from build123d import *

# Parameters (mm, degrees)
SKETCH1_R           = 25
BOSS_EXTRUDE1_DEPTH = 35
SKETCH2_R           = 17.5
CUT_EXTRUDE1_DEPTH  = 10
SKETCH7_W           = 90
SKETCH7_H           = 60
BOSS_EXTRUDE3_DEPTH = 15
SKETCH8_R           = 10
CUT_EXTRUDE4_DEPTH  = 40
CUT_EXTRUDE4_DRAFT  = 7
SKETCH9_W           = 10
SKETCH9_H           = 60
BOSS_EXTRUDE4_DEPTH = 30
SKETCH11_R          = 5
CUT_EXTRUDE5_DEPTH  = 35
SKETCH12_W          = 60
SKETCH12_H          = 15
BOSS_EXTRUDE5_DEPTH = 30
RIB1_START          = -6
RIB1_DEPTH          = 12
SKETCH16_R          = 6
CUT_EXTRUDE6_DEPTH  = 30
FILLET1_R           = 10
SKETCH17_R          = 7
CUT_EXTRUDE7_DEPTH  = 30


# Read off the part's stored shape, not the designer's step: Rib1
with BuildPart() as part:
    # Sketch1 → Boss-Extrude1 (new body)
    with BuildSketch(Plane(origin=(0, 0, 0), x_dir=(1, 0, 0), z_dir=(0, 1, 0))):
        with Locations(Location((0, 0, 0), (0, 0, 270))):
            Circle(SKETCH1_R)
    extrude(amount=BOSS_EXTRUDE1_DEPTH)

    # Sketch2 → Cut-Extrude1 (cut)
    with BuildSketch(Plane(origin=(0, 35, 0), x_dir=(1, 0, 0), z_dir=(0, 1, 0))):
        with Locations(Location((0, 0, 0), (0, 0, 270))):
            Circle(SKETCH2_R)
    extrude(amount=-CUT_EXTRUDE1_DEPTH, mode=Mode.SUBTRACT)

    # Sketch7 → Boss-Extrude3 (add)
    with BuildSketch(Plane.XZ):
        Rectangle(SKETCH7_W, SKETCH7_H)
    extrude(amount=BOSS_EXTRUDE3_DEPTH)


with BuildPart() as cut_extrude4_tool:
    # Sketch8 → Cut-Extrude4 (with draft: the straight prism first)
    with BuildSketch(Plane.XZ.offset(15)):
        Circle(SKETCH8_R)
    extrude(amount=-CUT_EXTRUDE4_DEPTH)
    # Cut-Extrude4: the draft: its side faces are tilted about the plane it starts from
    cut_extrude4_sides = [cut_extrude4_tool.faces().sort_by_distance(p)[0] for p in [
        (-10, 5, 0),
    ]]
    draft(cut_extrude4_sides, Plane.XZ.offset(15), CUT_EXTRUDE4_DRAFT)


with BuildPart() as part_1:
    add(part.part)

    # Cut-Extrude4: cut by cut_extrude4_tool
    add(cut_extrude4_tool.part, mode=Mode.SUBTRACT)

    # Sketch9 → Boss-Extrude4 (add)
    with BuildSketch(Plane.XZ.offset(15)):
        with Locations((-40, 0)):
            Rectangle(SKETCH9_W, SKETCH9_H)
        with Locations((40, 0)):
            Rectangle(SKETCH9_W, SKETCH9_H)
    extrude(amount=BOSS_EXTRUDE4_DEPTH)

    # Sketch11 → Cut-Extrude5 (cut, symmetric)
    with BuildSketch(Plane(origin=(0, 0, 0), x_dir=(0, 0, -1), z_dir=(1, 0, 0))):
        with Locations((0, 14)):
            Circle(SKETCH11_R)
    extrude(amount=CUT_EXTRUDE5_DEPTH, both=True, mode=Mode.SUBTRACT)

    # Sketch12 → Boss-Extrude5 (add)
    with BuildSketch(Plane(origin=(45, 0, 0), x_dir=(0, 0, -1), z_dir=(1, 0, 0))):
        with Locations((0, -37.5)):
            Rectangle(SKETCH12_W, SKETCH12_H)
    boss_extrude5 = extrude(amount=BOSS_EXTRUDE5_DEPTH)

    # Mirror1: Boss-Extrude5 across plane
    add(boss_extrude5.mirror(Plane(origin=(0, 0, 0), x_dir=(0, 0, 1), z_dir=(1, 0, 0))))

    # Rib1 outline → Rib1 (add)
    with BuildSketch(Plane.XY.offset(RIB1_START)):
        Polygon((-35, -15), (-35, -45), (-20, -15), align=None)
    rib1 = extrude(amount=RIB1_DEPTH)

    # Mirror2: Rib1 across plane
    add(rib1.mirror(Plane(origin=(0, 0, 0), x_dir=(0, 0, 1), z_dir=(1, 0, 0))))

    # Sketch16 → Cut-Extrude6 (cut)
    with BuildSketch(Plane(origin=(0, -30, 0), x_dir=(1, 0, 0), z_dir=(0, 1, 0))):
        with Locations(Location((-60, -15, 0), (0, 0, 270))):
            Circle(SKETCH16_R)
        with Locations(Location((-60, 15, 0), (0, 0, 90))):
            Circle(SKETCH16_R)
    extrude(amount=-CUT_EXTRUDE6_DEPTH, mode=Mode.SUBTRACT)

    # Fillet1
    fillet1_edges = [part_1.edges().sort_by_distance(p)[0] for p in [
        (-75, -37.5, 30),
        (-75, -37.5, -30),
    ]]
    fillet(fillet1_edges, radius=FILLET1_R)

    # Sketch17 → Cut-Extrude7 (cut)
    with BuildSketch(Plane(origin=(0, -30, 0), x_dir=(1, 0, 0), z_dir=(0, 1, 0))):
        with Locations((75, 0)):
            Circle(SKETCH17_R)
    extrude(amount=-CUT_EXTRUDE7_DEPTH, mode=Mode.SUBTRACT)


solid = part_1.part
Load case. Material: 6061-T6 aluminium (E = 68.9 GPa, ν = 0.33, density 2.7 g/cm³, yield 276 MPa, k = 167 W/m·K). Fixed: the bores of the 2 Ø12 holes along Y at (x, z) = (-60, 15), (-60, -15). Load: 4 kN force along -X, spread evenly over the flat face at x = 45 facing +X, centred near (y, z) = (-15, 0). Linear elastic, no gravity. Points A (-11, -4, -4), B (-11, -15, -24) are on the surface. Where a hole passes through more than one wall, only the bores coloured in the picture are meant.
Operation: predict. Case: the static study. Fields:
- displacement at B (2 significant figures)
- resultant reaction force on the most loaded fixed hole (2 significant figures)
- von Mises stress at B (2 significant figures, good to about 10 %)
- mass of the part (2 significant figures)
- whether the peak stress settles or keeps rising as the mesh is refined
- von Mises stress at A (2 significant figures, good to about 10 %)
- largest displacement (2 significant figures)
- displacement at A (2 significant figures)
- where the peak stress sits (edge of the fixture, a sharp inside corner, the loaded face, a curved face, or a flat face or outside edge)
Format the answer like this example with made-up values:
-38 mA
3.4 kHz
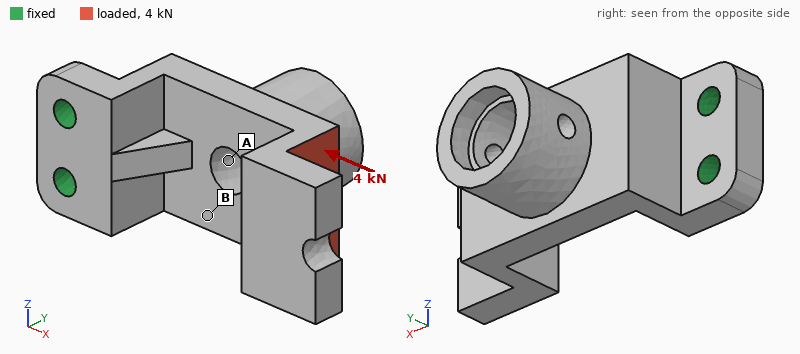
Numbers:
0.091 mm
2.0 kN
14 MPa
560 g
keeps rising
6.5 MPa
0.19 mm
0.10 mm
edge of the fixture
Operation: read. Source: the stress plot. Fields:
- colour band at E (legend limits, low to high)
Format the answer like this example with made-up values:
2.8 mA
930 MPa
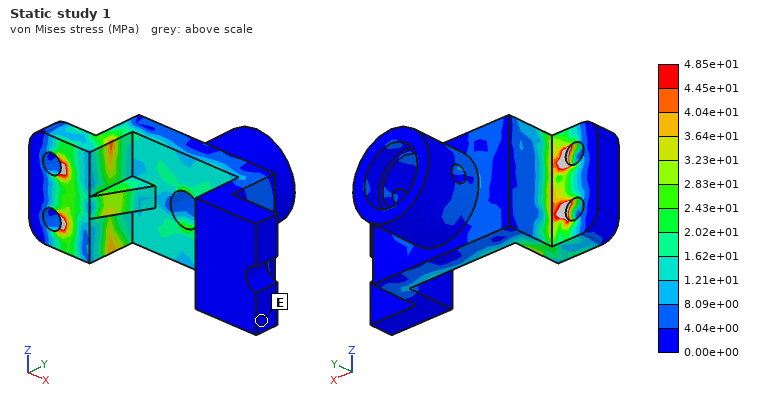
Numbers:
0.00e+00 to 4.04e+00 MPa
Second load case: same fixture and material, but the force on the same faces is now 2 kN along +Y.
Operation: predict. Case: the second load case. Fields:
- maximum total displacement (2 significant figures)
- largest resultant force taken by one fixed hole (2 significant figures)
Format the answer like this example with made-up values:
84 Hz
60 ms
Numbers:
1.2 mm
1.1 kN
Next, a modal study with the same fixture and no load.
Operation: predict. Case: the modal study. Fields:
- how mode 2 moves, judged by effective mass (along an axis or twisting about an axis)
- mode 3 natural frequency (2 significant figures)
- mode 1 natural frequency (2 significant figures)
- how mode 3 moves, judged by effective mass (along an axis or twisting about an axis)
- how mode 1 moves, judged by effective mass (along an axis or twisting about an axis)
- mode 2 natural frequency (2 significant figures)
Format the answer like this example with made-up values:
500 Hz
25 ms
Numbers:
along Z
2000 Hz
470 Hz
along X
along Y
860 Hz
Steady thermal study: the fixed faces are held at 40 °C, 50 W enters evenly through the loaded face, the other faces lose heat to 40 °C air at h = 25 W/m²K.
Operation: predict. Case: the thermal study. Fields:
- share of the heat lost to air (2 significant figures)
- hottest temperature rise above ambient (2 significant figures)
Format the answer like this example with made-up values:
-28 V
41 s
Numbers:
33 %
29 K
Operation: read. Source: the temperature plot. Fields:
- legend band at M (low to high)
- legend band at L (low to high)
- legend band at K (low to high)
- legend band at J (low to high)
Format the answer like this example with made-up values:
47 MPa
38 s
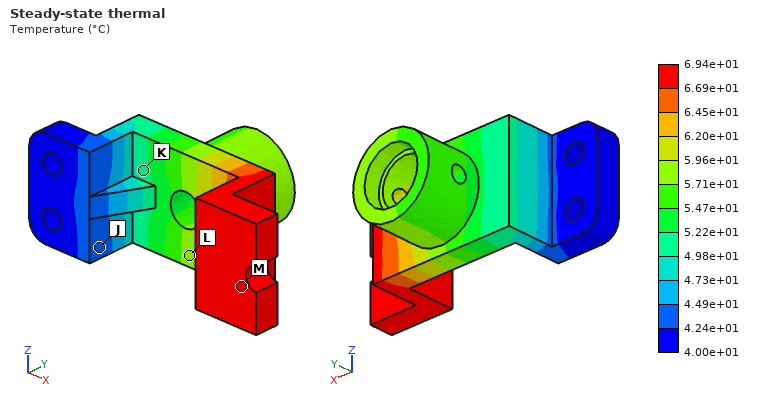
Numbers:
6.69e+01 to 6.94e+01 °C
5.71e+01 to 5.96e+01 °C
4.98e+01 to 5.22e+01 °C
4.24e+01 to 4.49e+01 °C
